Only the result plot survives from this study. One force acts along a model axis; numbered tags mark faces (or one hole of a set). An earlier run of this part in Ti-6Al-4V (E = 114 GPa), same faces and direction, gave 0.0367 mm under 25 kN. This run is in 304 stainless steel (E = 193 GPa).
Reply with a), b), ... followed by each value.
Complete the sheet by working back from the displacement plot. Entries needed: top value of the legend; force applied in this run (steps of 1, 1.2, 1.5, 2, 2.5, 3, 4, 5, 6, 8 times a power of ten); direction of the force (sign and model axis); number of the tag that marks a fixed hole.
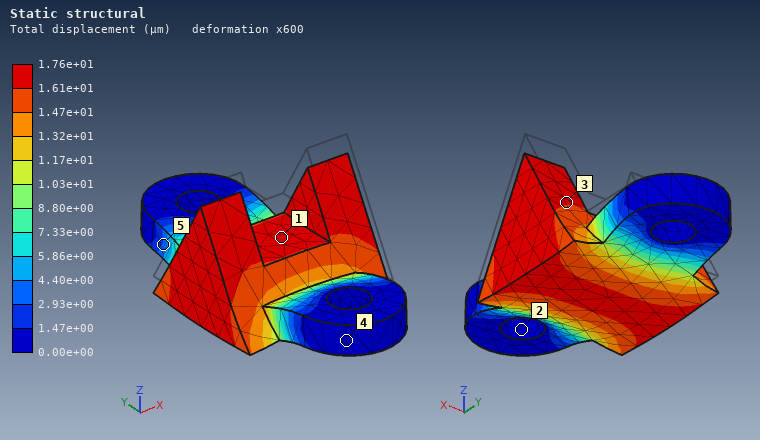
a) 1.76e+01 µm
b) 20 kN
c) -Z
d) 2
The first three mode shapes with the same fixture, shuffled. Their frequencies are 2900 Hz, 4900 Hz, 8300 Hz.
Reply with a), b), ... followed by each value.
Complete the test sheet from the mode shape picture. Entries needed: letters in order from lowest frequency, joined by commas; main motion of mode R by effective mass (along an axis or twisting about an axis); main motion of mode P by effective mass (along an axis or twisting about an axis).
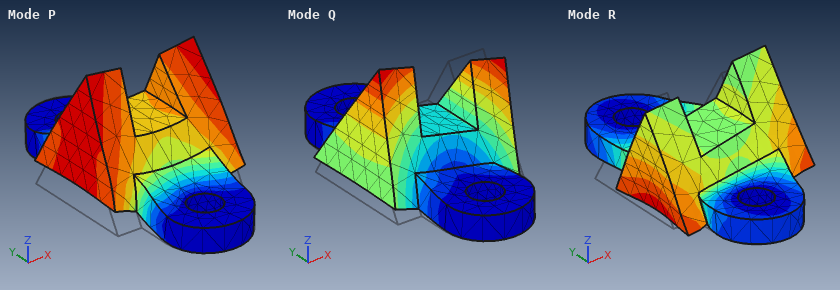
a) Q, P, R
b) along X
c) along Z
